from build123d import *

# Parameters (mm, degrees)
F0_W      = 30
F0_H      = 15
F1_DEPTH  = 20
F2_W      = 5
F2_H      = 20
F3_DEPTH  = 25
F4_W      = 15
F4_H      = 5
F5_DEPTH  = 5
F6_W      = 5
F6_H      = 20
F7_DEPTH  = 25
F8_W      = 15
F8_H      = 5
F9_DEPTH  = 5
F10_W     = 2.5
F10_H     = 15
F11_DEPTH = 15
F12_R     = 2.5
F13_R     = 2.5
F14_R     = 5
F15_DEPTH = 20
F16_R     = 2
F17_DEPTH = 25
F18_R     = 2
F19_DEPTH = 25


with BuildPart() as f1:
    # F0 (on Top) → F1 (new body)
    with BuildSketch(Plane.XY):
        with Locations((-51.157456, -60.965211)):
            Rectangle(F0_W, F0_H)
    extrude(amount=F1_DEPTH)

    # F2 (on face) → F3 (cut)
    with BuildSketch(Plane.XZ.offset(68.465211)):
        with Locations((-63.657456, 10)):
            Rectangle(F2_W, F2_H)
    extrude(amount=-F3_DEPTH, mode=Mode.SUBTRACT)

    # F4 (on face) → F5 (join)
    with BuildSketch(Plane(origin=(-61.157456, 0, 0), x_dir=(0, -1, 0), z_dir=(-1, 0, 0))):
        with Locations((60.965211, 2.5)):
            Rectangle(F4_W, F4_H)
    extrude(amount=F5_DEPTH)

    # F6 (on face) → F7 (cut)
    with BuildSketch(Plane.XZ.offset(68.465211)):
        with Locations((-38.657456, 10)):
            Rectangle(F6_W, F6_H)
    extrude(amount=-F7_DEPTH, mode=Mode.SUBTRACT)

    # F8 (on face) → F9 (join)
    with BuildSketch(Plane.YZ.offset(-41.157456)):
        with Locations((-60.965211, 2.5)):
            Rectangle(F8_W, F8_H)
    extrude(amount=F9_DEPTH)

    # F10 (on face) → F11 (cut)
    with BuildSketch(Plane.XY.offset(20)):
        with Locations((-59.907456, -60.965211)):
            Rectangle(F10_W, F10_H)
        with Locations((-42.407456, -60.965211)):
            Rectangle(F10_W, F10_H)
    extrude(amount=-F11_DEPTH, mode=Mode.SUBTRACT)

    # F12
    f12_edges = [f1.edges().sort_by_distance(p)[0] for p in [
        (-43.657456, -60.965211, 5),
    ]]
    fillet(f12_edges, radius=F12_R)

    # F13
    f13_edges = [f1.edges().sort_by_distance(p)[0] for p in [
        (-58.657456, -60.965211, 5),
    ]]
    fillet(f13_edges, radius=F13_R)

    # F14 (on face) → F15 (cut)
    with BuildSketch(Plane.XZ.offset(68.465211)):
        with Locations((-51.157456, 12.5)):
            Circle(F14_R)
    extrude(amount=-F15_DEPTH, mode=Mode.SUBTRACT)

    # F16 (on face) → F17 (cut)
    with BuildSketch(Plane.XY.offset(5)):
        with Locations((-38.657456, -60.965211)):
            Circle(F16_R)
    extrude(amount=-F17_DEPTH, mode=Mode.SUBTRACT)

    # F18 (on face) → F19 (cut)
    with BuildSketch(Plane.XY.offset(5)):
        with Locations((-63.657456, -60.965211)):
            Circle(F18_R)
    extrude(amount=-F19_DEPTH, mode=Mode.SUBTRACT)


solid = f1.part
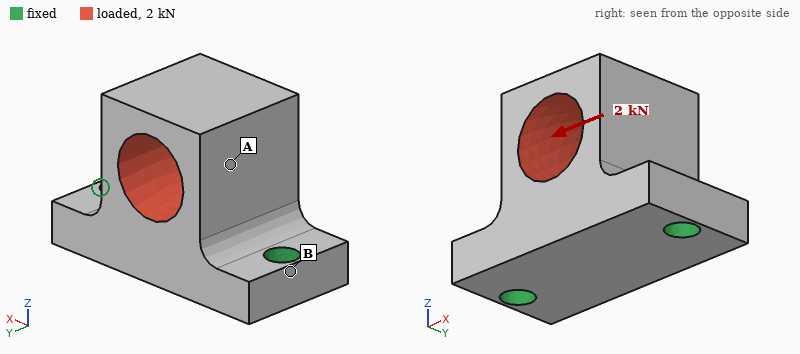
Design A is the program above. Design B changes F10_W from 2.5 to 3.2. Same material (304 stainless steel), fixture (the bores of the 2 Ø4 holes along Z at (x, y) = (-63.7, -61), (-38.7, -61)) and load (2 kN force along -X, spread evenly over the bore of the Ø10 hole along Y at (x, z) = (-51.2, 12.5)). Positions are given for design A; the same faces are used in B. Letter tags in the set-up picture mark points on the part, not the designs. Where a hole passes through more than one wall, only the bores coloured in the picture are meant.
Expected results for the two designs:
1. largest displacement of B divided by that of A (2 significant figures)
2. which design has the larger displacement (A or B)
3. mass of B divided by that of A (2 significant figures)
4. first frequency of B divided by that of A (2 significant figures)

1.2
B
0.96
1.0
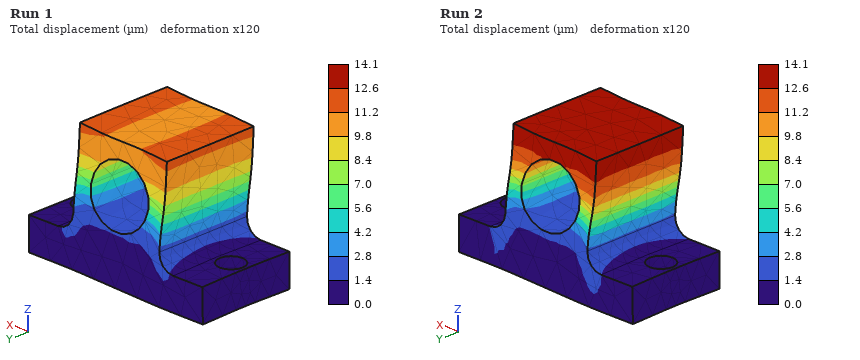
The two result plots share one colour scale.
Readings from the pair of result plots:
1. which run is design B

Run 2
